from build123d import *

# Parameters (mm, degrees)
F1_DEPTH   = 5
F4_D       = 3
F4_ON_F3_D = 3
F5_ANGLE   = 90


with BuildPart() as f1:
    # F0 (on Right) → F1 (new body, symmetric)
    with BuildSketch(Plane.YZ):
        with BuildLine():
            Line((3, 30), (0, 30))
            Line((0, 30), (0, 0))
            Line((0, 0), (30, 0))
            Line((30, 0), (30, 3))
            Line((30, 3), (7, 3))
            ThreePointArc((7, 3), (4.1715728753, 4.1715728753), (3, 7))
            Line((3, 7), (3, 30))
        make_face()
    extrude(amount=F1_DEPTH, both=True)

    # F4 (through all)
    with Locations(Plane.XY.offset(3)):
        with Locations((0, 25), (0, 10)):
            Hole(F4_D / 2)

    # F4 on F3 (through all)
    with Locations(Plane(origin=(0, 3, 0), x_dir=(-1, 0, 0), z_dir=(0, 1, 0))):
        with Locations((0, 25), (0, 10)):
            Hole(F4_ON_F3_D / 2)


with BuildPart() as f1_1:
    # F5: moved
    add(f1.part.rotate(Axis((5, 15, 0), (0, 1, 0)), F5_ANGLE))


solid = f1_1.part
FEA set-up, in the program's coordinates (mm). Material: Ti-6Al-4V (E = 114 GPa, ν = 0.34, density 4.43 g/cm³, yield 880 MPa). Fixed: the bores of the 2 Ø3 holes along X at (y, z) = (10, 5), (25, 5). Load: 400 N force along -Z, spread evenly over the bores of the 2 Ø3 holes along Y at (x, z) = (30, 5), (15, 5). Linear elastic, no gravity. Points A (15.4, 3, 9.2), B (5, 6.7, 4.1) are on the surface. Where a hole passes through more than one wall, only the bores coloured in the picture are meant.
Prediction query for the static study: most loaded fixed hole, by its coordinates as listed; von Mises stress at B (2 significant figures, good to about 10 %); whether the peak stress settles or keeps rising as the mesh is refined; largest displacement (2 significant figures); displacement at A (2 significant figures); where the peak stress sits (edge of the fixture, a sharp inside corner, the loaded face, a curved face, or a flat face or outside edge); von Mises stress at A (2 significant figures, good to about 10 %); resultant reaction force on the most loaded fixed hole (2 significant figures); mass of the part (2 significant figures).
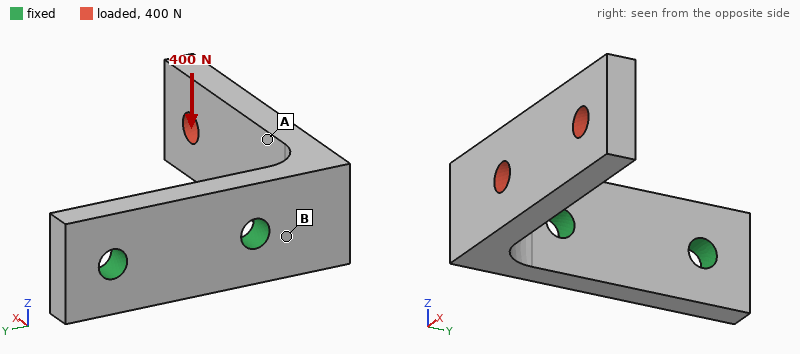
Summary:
(10, 5)
230 MPa
keeps rising
0.30 mm
0.099 mm
edge of the fixture
64 MPa
510 N
7.4 g
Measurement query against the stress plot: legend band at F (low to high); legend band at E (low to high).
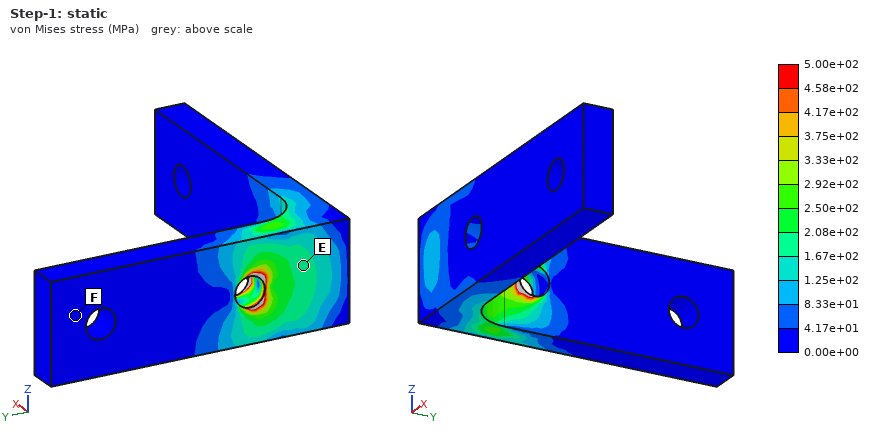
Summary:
0.00e+00 to 4.17e+01 MPa
1.67e+02 to 2.08e+02 MPa
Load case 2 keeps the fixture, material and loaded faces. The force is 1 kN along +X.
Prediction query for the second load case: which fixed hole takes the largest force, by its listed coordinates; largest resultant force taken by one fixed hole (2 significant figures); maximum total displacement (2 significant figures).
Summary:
(10, 5)
1.1 kN
0.33 mm
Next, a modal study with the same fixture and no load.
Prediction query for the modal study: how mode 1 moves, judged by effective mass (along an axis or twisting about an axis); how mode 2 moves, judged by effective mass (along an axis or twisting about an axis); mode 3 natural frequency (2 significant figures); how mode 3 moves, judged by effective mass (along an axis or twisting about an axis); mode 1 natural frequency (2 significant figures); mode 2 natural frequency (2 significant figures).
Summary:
along Y
along Z
11 kHz
along X
2500 Hz
4000 Hz
